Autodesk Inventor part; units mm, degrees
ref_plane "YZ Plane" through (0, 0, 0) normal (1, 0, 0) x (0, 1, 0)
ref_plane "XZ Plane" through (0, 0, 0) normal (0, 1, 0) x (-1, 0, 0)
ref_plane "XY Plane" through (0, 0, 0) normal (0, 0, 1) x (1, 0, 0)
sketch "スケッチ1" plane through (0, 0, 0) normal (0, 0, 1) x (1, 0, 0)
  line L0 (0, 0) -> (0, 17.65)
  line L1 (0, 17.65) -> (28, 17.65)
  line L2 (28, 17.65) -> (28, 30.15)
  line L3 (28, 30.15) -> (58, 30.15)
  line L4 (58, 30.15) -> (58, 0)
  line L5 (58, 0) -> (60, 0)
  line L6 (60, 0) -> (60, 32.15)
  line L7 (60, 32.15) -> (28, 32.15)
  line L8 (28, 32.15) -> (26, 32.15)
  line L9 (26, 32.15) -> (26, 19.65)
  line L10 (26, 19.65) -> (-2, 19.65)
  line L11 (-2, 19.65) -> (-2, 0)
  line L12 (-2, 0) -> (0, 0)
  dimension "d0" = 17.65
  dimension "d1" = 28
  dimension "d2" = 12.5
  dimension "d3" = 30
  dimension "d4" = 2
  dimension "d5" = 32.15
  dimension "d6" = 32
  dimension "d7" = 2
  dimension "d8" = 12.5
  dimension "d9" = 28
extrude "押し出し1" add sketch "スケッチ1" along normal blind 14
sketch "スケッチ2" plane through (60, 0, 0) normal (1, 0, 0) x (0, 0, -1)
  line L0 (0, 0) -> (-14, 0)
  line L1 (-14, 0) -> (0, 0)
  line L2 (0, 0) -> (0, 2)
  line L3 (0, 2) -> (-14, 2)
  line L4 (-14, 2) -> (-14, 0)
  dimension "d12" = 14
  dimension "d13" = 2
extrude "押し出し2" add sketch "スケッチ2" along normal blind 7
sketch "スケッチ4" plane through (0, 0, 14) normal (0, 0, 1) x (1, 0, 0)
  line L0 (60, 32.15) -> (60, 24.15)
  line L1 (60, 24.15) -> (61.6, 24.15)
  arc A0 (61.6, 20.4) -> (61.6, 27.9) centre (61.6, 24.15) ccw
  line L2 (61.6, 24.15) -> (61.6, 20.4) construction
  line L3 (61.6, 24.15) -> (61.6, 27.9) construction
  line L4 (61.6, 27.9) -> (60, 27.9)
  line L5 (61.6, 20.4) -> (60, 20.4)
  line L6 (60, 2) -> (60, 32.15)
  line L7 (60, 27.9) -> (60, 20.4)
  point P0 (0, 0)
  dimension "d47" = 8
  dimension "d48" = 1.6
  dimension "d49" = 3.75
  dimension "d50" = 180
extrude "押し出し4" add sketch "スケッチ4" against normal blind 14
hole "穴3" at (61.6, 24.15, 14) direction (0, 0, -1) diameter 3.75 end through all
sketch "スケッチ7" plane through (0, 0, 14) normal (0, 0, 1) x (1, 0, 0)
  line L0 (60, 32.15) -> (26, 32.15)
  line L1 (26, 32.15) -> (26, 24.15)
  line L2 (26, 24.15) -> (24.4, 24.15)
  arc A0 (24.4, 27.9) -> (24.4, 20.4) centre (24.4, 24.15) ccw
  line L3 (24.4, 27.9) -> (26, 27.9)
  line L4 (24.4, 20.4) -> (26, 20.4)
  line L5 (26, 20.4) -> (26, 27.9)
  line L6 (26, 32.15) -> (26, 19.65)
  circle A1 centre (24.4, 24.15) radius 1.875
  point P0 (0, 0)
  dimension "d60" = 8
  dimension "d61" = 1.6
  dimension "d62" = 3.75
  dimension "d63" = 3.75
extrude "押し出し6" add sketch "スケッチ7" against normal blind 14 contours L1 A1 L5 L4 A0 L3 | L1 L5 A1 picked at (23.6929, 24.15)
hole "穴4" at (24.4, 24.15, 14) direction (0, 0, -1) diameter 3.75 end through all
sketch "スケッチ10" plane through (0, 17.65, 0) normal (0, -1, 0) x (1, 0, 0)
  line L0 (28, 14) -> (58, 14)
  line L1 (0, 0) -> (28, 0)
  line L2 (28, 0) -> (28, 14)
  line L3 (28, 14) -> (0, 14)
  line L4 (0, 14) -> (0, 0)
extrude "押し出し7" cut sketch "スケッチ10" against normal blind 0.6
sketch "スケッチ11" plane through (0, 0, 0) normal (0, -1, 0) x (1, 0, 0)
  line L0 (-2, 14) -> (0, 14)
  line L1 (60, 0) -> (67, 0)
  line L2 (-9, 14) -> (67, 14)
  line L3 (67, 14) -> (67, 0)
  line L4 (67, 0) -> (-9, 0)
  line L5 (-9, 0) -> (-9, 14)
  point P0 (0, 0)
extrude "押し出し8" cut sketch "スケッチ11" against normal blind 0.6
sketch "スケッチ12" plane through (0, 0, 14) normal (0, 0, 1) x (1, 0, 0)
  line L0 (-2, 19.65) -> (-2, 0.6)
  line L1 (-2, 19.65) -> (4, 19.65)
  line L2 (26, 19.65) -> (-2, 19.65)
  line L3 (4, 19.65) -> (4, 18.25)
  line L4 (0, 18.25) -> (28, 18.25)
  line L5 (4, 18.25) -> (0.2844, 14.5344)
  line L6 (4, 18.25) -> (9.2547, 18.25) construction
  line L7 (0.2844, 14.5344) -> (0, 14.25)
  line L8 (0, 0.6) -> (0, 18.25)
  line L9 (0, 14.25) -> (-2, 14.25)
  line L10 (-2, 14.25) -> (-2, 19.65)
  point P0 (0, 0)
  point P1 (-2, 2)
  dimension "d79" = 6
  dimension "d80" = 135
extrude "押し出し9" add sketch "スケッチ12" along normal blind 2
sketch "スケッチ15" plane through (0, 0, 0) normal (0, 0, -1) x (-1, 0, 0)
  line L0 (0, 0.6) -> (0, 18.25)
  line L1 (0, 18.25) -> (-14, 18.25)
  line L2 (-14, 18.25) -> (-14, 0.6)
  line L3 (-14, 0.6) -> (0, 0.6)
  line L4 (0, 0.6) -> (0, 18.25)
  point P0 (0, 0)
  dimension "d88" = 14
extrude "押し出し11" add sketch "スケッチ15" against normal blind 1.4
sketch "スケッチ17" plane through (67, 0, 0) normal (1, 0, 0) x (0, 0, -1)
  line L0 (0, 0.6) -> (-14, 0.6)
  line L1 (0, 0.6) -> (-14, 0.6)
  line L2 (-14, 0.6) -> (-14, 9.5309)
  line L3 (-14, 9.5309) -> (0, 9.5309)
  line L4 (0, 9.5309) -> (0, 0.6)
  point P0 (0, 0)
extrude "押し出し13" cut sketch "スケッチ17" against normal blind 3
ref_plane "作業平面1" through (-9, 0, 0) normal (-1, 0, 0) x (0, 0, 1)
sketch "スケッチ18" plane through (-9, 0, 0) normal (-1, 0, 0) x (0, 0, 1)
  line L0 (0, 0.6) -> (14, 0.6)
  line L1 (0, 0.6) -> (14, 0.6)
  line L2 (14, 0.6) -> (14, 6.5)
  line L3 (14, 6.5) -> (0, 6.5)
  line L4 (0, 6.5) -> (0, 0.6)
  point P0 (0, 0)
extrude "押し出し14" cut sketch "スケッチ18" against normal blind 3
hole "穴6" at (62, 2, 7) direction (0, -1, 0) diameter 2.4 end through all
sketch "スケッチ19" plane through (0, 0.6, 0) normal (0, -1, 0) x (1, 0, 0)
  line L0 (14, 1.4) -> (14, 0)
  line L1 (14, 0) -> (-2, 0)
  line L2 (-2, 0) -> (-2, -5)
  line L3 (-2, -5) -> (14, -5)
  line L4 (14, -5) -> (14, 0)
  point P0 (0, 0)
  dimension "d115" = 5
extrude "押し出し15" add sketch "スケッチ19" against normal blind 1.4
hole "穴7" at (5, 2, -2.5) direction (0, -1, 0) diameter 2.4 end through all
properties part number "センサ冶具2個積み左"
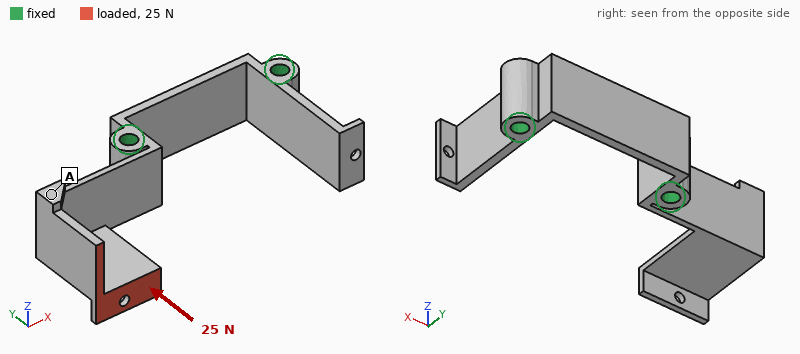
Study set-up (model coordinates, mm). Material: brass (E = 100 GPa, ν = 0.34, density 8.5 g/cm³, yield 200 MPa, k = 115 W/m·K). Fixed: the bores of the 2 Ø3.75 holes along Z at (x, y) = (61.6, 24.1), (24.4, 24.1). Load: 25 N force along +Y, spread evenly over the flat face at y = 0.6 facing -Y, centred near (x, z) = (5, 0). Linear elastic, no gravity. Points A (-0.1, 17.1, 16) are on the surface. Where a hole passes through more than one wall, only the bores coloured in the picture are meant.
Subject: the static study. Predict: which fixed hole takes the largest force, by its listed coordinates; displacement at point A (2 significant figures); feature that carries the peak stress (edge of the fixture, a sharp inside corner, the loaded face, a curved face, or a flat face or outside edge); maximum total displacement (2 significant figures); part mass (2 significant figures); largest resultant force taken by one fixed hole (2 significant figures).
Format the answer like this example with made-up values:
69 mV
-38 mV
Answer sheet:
(24.4, 24.1)
0.32 mm
a flat face or outside edge
0.60 mm
37 g
25 N
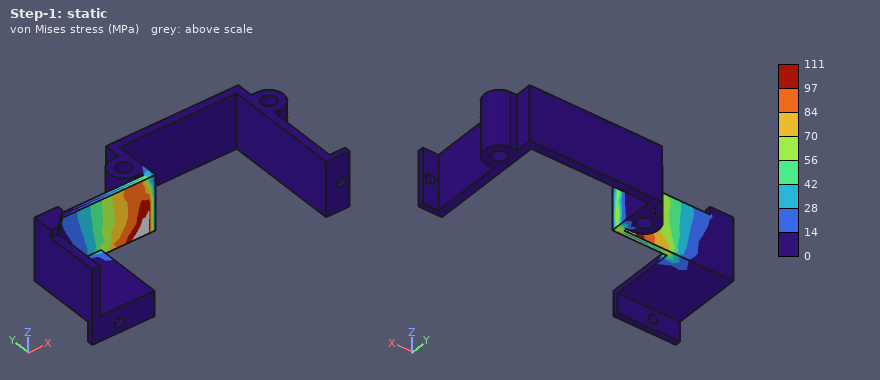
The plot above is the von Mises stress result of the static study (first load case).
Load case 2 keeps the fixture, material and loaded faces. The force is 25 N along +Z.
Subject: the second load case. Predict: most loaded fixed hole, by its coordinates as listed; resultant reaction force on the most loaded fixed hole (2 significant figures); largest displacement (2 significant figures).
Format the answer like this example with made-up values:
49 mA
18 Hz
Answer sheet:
(24.4, 24.1)
25 N
0.36 mm
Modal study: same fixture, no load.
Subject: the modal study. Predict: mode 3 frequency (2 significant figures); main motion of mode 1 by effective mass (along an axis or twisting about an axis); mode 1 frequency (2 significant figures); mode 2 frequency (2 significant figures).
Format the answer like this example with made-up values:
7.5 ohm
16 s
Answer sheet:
2100 Hz
along Y
340 Hz
740 Hz
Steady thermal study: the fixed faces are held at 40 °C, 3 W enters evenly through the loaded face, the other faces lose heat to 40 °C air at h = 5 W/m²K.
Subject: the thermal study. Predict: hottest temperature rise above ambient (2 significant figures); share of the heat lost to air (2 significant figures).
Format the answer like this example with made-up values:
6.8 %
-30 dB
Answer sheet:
40 K
9.0 %
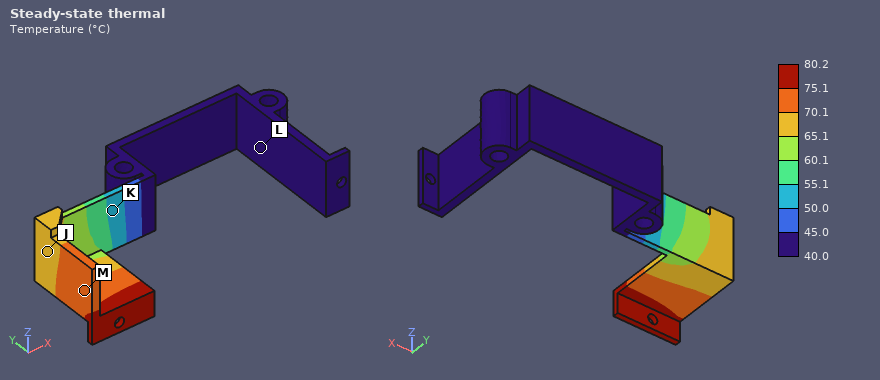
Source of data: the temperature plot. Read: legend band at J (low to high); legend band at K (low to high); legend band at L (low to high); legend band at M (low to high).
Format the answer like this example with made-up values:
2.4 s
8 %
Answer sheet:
65.1 to 70.1 °C
50.0 to 55.1 °C
40.0 to 45.0 °C
70.1 to 75.1 °C
